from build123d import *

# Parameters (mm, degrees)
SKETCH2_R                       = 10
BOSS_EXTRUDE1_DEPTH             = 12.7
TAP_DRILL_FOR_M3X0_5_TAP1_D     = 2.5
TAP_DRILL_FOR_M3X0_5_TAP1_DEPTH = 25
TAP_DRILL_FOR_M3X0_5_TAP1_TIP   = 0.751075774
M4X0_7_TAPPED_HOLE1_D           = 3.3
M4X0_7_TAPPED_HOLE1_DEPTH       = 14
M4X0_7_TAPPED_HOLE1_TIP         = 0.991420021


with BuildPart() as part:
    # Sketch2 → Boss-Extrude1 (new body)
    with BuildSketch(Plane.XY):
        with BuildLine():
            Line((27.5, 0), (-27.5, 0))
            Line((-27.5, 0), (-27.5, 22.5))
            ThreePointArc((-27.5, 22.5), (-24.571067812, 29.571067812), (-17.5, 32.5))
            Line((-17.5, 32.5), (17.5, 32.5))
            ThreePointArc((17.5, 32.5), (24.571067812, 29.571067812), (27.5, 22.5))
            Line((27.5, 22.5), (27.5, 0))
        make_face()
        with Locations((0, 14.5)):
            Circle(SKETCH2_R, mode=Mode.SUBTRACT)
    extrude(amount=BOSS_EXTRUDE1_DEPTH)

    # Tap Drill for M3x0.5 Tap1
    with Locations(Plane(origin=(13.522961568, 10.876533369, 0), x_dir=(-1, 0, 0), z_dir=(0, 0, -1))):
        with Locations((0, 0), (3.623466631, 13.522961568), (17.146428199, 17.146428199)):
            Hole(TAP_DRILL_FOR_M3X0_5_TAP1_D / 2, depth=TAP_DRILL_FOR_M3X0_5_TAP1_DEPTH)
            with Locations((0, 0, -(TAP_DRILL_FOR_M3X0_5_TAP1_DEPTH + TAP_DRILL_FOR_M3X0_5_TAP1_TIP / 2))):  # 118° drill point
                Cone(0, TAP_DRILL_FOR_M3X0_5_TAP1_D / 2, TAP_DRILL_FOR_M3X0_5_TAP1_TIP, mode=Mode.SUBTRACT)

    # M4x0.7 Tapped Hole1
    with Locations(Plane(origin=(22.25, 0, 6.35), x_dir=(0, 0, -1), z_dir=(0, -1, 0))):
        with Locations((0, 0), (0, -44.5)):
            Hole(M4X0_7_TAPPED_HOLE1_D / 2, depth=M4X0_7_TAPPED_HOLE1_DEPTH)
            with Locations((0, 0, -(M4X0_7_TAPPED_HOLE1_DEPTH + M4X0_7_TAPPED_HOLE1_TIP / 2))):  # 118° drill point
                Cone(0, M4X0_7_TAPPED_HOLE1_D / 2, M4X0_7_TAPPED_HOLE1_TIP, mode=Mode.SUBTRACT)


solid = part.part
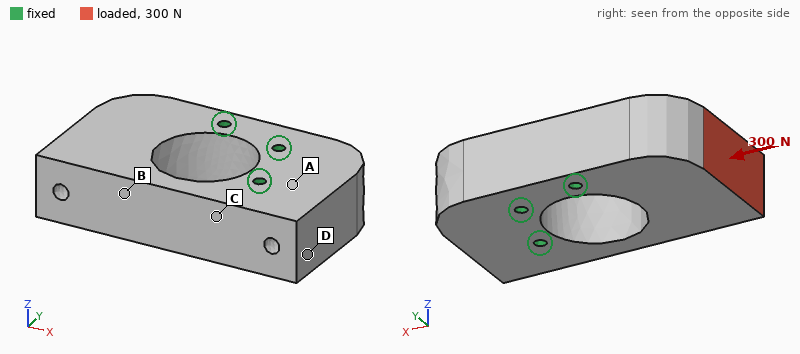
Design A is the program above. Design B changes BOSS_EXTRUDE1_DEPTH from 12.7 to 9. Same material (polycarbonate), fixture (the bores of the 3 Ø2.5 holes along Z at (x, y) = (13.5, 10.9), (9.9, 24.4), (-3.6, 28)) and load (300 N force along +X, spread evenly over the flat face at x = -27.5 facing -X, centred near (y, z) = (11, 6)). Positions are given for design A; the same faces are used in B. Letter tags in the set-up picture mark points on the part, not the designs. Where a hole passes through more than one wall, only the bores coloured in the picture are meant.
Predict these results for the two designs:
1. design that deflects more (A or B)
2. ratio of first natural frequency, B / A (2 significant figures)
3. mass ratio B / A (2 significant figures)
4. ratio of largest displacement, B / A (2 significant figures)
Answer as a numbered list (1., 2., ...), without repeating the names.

1. B
2. 0.77
3. 0.70
4. 1.4
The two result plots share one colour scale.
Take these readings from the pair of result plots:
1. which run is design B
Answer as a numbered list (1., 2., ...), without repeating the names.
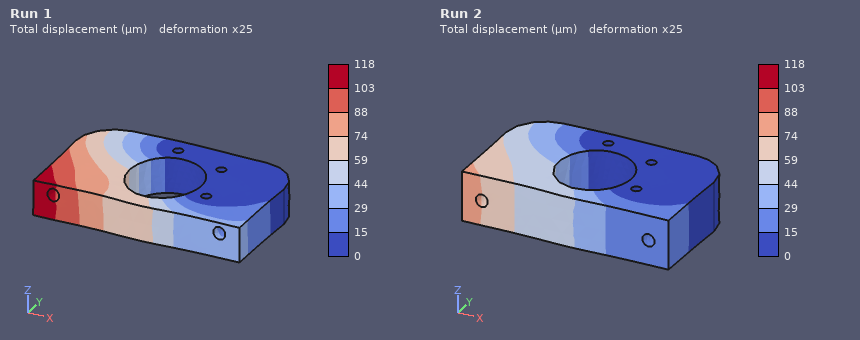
1. Run 1
